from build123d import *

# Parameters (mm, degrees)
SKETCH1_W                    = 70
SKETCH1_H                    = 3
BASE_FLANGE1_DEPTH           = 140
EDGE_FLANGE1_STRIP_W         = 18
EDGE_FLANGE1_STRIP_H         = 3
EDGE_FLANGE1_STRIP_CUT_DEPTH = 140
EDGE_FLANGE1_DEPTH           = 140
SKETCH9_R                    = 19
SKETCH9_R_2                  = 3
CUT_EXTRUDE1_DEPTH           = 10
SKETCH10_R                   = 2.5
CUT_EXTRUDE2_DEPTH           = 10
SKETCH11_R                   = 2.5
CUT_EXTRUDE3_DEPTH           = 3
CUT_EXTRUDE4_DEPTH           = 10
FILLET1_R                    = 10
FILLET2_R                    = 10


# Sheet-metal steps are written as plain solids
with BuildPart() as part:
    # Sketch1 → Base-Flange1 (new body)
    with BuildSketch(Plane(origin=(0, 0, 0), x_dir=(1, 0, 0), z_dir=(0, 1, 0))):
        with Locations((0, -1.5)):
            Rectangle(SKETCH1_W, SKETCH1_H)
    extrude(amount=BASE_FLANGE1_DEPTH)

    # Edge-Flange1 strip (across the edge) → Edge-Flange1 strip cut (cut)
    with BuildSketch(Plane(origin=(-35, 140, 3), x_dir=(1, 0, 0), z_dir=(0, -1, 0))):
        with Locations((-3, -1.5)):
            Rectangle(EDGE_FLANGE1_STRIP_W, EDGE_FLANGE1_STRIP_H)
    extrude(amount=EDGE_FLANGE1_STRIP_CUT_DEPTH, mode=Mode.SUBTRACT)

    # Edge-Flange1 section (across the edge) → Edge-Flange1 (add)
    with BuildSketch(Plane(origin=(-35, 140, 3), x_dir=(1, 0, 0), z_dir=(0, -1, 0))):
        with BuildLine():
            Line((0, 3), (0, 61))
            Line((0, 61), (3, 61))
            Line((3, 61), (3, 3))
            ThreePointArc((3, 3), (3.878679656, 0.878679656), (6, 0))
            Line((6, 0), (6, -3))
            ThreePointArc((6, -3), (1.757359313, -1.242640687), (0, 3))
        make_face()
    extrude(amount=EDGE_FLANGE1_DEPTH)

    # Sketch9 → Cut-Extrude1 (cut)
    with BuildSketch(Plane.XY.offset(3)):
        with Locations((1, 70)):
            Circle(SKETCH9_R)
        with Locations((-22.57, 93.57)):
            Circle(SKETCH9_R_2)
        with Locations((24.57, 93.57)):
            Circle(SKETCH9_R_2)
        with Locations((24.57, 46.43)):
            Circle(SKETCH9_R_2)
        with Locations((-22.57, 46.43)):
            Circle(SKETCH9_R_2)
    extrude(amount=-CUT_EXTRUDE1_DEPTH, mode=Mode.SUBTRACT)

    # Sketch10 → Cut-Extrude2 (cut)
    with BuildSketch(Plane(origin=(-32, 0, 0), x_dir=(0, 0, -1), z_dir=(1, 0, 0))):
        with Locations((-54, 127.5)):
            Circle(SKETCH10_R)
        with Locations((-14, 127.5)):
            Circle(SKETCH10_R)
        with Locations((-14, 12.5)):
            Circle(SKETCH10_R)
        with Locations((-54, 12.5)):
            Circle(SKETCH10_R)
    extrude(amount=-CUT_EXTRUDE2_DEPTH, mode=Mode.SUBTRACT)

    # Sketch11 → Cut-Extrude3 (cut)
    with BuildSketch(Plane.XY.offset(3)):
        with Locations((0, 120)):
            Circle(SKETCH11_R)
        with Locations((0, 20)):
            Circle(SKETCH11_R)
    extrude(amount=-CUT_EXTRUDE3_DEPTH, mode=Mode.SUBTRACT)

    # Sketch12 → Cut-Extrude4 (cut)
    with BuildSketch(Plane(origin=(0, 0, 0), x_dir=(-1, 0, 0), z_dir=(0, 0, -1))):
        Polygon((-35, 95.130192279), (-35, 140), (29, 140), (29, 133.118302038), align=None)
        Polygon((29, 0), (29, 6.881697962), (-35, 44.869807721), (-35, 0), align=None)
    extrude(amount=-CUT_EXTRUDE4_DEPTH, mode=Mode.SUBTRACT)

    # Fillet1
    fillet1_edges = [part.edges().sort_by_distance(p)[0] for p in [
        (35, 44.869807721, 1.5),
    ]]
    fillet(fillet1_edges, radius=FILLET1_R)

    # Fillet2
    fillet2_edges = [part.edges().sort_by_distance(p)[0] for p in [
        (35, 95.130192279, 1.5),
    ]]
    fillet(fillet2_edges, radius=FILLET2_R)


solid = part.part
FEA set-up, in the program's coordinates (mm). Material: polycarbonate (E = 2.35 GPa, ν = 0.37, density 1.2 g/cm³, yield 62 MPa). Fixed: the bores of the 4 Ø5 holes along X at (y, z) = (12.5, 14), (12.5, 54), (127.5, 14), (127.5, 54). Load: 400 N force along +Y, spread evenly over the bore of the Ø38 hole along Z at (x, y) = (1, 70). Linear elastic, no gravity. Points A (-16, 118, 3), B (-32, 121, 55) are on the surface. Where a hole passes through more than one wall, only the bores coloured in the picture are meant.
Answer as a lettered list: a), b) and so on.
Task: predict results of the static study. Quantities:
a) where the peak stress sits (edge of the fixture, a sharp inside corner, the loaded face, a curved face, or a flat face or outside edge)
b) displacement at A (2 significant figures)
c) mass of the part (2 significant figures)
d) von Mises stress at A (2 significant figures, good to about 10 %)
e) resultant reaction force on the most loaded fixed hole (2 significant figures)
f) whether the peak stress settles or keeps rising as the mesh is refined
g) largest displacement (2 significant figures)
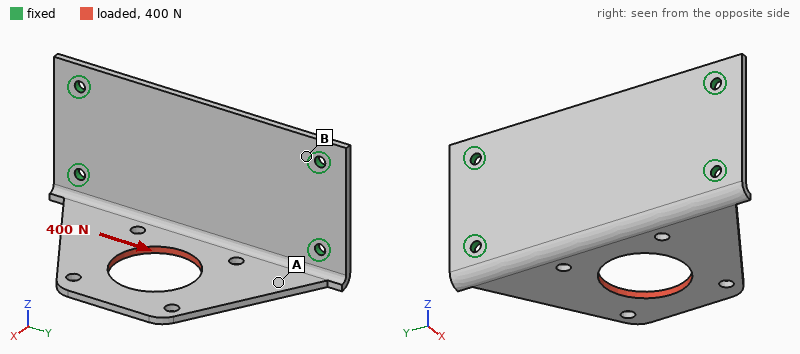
a) edge of the fixture
b) 0.59 mm
c) 48 g
d) 5.4 MPa
e) 210 N
f) keeps rising
g) 0.93 mm
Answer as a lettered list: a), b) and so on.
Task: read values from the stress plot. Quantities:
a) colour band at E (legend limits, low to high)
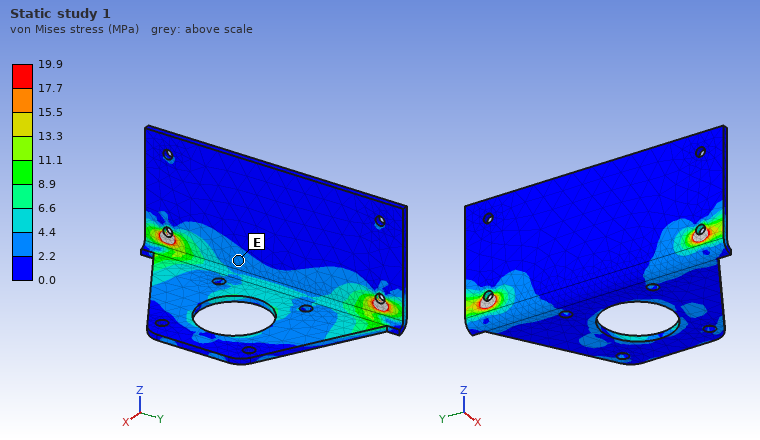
a) 2.2 to 4.4 MPa
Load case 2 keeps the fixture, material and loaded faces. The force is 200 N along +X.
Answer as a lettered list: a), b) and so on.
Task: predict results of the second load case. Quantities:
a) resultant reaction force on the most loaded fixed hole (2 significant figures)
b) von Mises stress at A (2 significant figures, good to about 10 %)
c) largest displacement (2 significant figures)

a) 130 N
b) 3.1 MPa
c) 1.9 mm
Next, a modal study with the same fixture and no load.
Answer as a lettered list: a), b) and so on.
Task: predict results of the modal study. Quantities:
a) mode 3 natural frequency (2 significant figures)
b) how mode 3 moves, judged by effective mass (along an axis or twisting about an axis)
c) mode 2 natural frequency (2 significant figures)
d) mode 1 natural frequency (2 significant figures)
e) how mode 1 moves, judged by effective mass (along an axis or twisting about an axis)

a) 410 Hz
b) along X
c) 360 Hz
d) 140 Hz
e) along Z
